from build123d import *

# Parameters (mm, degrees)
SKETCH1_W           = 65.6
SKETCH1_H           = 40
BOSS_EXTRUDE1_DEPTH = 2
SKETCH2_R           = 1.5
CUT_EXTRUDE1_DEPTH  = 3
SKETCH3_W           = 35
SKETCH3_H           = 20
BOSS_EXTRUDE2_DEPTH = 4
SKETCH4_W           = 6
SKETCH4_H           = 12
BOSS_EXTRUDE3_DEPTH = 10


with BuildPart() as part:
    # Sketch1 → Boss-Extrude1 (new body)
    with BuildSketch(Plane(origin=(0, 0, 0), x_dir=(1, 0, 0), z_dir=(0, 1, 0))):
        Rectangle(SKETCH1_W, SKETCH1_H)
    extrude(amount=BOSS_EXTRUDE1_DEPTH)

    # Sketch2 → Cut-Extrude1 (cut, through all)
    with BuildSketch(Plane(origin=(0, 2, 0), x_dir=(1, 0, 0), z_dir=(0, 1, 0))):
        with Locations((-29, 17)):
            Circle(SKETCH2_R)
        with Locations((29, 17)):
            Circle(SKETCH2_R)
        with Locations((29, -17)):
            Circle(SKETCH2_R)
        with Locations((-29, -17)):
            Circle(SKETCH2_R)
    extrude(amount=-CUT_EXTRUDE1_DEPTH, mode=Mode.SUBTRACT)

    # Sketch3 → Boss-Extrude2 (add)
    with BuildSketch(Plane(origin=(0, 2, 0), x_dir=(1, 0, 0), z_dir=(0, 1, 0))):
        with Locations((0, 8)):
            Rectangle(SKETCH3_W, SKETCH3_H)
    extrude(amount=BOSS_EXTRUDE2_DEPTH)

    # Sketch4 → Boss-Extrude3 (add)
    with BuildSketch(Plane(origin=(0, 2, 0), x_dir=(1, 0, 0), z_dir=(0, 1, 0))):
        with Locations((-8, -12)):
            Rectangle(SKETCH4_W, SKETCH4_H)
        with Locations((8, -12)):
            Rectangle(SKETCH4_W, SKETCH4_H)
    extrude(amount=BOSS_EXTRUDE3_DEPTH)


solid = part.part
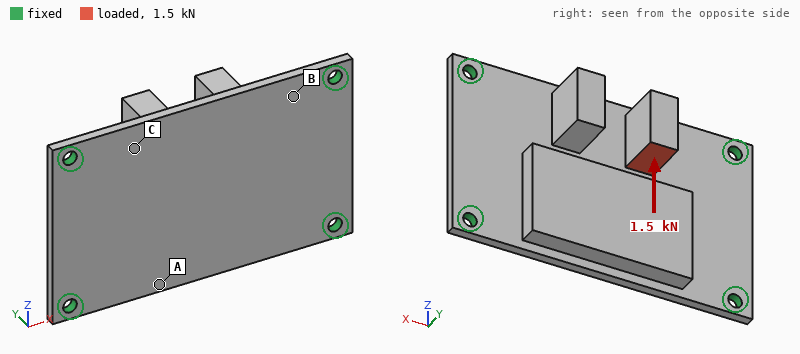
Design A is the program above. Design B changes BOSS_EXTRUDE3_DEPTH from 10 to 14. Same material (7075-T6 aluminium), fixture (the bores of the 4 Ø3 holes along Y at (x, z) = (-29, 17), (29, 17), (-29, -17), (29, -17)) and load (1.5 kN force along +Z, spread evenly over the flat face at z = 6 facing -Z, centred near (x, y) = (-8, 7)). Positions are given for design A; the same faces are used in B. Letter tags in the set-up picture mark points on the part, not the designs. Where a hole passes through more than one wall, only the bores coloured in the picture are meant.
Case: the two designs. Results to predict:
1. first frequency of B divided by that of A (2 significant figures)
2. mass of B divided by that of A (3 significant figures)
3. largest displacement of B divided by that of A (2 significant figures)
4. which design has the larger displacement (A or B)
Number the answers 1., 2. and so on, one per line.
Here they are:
1. 0.91
2. 1.06
3. 1.6
4. B
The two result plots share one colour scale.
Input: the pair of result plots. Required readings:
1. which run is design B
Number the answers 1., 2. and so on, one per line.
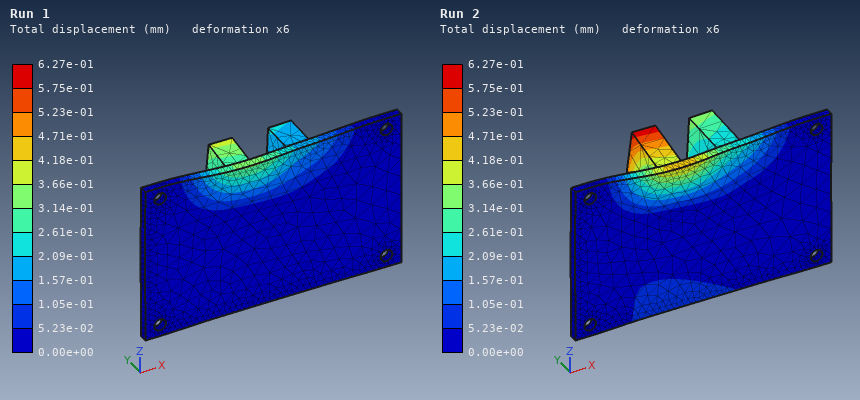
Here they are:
1. Run 2
